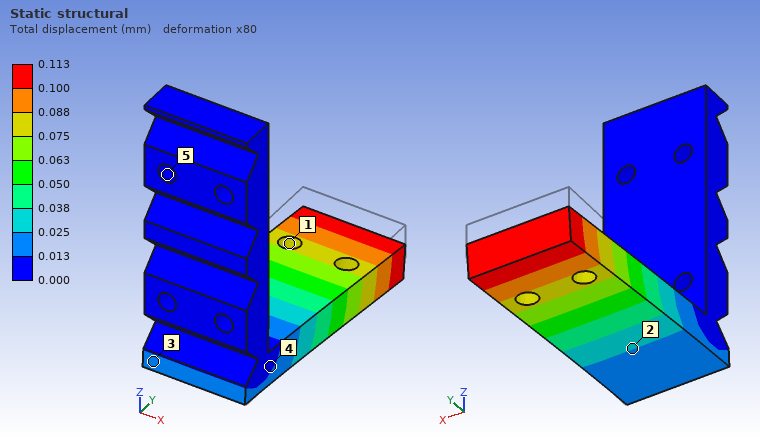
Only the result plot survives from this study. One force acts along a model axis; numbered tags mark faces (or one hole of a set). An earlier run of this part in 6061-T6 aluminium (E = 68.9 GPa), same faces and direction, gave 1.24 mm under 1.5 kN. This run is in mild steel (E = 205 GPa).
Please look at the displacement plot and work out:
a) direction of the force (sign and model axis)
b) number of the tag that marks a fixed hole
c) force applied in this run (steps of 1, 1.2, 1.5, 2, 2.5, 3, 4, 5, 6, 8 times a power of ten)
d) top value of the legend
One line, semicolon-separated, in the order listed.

-Z; 5; 400 N; 0.113 mm
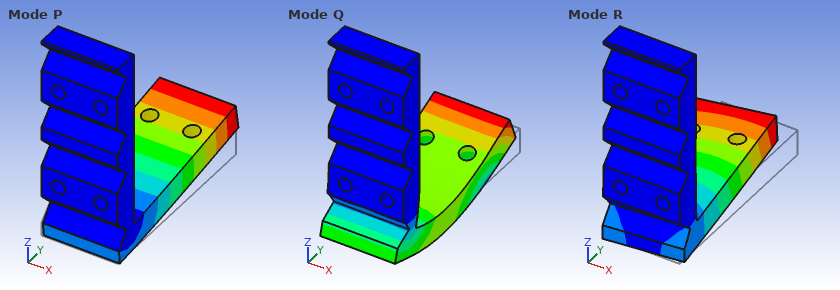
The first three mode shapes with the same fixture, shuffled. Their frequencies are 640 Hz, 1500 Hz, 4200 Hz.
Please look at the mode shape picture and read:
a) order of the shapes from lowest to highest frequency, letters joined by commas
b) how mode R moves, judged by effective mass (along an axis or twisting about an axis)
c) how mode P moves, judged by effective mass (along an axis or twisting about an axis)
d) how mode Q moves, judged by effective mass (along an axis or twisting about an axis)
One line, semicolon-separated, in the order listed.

P, R, Q; along X; along Z; along Y
